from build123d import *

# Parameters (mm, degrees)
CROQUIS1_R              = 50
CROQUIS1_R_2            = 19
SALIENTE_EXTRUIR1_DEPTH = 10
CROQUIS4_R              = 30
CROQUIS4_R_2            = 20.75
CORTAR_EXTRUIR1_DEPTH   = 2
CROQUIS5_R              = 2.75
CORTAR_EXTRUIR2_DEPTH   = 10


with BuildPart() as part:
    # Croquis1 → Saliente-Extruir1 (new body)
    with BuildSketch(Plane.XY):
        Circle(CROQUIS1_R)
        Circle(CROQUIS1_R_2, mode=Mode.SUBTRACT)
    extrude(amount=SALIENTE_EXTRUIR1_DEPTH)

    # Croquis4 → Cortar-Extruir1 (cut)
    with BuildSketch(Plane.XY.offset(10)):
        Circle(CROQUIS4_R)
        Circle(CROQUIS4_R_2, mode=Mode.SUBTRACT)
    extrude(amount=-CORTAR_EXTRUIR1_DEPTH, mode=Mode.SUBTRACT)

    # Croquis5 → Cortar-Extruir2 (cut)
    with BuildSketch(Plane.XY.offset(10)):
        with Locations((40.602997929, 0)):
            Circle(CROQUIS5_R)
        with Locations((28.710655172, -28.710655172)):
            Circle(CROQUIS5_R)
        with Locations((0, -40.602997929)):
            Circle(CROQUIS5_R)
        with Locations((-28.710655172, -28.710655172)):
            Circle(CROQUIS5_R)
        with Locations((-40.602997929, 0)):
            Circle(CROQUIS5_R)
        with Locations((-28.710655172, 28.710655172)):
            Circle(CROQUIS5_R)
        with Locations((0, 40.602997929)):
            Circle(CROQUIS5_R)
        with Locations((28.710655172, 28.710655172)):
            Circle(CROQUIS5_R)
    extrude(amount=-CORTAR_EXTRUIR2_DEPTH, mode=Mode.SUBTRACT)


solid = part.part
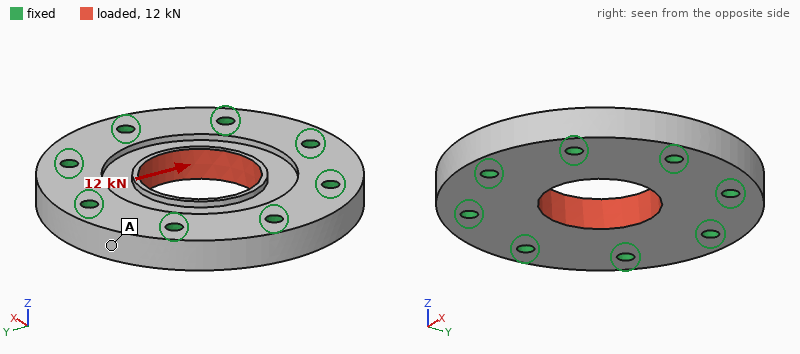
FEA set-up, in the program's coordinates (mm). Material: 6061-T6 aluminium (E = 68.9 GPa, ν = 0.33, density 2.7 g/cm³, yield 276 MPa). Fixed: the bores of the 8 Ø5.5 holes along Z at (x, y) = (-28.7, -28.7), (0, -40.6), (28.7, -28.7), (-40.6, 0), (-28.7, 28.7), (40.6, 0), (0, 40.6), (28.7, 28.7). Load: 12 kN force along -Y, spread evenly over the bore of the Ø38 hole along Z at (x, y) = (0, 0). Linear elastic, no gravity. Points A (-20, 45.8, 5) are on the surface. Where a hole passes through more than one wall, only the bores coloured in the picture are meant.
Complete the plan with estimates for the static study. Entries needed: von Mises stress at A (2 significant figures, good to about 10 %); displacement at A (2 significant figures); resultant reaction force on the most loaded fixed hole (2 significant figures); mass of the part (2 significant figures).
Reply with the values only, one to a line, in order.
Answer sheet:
5.2 MPa
1.5 µm
2.3 kN
170 g
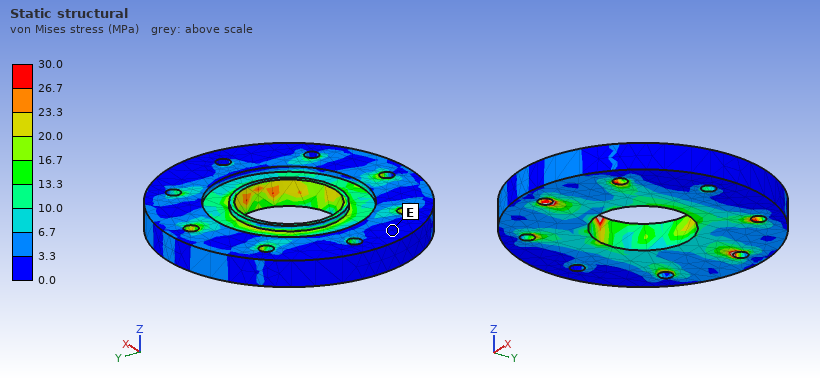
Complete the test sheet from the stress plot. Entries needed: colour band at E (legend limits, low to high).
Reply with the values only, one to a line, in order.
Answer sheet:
0.0 to 3.3 MPa
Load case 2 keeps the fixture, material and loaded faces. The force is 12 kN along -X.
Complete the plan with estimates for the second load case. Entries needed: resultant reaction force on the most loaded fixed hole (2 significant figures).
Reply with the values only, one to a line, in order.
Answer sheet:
2.3 kN
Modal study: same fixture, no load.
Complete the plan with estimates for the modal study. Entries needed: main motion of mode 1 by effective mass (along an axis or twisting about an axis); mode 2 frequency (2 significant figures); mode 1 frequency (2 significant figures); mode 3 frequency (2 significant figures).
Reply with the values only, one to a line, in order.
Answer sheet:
along Z
21 kHz
17 kHz
21 kHz
